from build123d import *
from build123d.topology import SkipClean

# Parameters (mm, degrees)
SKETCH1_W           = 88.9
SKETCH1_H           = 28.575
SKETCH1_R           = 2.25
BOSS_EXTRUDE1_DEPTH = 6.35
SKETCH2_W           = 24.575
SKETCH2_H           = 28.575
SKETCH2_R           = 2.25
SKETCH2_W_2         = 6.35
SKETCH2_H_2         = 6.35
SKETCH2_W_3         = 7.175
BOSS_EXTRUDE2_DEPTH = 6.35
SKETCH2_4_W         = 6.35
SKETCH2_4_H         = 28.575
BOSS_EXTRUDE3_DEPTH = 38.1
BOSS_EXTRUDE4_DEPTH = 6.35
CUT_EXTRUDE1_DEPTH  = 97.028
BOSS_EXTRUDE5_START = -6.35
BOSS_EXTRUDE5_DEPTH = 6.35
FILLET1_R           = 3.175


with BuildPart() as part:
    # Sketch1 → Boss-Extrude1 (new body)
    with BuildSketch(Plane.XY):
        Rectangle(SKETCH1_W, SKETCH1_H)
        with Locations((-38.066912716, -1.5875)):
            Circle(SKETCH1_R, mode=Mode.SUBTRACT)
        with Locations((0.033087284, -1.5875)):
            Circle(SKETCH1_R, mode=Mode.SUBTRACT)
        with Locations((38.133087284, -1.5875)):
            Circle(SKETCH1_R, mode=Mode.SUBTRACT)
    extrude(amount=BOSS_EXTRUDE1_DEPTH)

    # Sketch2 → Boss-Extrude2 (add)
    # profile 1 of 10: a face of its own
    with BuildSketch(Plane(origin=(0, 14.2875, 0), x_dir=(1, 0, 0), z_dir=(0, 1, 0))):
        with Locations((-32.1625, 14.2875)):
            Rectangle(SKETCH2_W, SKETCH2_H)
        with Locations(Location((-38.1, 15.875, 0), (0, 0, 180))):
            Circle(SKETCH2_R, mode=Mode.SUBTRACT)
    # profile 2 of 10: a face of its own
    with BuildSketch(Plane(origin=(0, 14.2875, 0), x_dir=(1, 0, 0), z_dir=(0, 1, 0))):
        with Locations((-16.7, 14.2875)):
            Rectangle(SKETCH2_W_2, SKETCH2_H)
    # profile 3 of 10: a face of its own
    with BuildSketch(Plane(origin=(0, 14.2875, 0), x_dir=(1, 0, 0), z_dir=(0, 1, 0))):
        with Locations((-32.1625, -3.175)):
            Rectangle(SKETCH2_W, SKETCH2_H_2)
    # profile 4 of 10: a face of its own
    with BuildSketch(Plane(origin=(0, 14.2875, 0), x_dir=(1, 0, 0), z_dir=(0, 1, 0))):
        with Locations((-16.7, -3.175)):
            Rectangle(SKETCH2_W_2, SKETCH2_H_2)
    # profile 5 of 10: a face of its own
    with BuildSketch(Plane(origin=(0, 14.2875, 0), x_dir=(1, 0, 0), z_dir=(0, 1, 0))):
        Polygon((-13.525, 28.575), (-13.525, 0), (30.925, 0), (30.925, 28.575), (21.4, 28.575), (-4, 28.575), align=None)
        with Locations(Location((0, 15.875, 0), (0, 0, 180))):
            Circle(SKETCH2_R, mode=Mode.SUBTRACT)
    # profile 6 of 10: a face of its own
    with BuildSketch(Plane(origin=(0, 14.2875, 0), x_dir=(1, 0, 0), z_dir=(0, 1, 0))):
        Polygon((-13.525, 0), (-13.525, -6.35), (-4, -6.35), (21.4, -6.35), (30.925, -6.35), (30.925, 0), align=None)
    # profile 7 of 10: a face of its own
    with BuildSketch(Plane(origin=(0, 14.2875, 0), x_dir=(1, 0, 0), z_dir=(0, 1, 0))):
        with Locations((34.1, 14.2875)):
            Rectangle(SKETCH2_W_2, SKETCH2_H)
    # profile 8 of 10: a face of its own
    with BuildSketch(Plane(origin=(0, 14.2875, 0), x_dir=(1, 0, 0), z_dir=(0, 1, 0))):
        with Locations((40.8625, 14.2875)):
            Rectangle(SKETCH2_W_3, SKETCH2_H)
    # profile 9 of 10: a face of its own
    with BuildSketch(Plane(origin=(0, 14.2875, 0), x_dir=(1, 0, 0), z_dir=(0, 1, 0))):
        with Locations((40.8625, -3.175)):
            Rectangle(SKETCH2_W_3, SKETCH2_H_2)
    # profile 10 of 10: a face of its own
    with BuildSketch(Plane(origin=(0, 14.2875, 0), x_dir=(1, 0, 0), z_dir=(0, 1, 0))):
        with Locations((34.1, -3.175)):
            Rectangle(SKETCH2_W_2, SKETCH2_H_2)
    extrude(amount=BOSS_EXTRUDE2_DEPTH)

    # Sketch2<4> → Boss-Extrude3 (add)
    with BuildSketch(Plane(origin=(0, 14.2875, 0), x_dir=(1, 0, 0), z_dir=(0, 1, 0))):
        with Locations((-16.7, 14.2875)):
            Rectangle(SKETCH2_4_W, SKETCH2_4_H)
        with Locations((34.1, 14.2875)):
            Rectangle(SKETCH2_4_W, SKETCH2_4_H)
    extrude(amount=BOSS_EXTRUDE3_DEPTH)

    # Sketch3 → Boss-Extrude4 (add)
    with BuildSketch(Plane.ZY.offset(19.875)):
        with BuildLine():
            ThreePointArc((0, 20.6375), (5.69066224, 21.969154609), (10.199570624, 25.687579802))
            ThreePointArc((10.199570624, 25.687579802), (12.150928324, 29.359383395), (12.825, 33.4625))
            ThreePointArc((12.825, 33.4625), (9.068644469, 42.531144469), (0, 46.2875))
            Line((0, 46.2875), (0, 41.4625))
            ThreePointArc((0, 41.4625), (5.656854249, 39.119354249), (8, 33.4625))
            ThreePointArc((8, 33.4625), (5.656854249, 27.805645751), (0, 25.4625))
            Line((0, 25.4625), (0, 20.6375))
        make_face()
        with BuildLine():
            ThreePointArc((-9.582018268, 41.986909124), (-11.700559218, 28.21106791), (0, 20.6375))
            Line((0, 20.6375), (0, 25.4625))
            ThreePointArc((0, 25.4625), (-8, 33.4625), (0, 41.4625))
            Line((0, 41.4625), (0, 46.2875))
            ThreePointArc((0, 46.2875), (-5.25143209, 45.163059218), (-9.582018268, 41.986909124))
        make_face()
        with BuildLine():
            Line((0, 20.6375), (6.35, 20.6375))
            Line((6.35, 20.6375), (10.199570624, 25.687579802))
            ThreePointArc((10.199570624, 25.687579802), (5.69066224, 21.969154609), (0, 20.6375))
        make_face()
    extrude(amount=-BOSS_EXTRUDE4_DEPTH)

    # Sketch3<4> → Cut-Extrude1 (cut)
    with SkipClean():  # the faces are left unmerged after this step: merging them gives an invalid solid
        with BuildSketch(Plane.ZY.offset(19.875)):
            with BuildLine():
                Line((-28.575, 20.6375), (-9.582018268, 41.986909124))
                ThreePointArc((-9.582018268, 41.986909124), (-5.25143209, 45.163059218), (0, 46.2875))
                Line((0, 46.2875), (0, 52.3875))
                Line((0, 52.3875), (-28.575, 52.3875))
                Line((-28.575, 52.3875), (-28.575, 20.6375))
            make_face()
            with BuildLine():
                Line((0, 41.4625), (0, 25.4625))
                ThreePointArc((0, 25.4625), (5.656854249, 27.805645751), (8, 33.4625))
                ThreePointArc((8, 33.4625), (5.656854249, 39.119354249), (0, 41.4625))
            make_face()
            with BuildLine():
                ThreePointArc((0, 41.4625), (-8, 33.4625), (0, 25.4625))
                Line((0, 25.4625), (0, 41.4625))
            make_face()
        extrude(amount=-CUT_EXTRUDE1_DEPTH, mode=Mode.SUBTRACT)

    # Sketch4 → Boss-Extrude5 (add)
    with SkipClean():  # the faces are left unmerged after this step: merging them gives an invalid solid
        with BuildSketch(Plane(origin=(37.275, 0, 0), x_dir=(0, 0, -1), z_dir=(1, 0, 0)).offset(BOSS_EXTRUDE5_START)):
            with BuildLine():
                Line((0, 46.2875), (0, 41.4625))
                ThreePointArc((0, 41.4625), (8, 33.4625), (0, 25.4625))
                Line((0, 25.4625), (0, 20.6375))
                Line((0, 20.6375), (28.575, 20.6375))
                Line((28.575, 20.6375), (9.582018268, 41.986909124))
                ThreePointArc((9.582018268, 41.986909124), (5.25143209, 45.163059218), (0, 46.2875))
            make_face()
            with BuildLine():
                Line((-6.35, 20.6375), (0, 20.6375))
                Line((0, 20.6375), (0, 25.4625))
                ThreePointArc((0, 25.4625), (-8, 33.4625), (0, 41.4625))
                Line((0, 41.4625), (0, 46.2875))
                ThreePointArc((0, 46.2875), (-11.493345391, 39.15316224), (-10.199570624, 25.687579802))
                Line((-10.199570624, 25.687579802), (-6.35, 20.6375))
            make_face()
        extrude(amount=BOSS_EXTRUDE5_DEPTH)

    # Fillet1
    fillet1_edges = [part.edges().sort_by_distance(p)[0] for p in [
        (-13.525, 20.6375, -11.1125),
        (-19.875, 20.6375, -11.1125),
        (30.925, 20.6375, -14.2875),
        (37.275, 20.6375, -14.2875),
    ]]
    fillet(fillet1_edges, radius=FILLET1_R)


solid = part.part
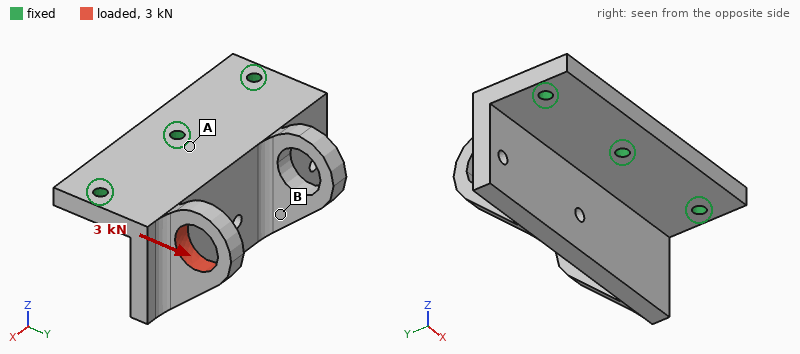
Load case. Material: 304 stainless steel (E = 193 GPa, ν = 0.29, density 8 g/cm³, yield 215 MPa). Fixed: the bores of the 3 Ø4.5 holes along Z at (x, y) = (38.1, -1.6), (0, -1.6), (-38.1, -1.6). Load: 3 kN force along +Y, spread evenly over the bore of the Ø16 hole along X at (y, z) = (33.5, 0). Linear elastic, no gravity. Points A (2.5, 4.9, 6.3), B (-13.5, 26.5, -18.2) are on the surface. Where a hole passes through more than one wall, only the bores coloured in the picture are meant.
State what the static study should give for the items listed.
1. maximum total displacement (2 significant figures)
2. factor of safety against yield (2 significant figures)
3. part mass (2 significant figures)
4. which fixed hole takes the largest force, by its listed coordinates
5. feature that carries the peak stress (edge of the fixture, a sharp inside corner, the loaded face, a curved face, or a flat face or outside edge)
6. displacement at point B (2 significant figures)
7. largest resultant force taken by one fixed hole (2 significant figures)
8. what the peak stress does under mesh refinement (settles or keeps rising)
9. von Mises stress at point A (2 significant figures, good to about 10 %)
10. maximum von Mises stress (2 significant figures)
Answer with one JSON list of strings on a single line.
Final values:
["37 µm", "1.5", "340 g", "(38.1, -1.6)", "a curved face", "12 µm", "2.6 kN", "settles", "15 MPa", "140 MPa"]
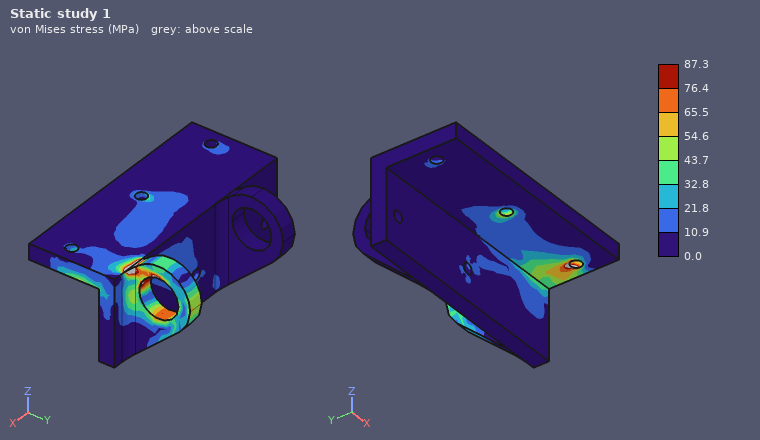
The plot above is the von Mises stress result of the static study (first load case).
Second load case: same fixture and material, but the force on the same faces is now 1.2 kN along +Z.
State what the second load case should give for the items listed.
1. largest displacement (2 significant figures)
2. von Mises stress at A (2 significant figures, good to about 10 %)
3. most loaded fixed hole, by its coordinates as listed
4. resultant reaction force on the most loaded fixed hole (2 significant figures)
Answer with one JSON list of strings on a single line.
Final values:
["0.13 mm", "70 MPa", "(38.1, -1.6)", "910 N"]
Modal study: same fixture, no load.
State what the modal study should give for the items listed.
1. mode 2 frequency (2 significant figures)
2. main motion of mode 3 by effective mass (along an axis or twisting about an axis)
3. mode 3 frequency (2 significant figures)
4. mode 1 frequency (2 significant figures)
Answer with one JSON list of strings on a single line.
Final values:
["3200 Hz", "along X", "6400 Hz", "1900 Hz"]
